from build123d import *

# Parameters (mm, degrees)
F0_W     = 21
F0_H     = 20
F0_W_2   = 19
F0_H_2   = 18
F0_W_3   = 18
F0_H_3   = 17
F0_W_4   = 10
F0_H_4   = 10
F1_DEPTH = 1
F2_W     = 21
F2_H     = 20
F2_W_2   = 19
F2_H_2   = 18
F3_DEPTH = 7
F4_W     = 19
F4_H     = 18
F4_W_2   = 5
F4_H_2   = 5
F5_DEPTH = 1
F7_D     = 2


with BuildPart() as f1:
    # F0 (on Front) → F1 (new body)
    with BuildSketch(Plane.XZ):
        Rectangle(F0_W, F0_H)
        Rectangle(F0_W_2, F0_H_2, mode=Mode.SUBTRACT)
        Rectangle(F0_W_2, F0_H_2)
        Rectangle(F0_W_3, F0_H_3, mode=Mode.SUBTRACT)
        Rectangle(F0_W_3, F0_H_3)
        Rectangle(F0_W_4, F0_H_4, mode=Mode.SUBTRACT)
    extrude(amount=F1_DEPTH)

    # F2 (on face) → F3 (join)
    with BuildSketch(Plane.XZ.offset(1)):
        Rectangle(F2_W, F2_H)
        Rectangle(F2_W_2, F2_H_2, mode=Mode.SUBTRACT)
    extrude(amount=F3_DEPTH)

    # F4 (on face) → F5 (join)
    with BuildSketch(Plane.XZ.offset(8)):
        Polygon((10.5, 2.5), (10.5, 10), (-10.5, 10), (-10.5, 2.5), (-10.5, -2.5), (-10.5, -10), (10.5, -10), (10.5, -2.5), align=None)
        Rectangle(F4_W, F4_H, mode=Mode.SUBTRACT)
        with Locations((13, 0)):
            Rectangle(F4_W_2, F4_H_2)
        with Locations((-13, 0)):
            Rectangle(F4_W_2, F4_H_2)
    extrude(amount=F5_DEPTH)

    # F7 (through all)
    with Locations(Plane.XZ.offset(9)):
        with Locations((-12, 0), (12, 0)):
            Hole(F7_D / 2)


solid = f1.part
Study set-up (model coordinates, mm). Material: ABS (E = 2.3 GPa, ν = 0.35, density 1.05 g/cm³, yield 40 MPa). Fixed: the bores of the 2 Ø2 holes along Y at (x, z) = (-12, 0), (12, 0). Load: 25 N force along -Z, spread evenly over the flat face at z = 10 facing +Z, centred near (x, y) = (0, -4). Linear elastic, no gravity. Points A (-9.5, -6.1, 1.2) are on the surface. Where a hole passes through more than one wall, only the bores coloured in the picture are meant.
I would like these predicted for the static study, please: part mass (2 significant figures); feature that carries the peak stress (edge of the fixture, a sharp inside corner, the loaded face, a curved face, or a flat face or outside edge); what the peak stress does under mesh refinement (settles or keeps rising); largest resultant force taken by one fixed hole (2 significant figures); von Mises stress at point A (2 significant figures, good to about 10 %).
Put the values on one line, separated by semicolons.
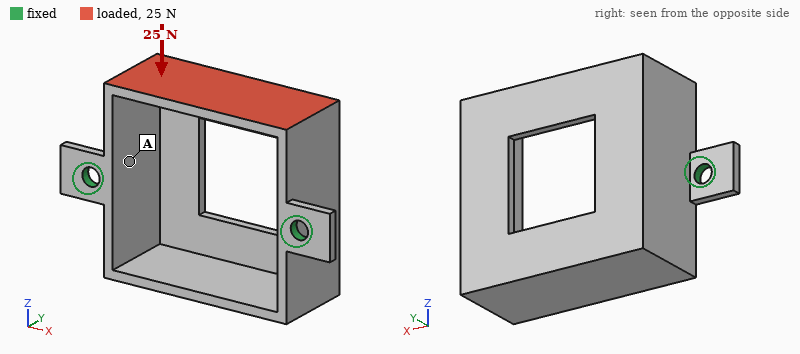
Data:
1.0 g; edge of the fixture; keeps rising; 13 N; 4.1 MPa
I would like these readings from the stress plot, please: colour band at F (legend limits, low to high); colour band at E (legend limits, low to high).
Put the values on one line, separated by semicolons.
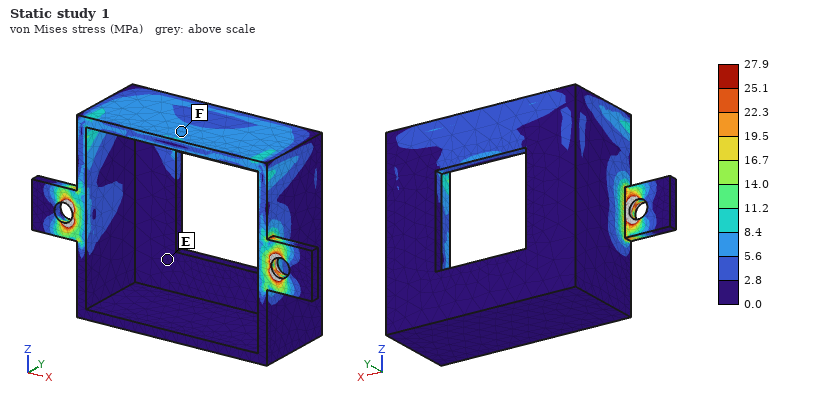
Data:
5.6 to 8.4 MPa; 0.0 to 2.8 MPa
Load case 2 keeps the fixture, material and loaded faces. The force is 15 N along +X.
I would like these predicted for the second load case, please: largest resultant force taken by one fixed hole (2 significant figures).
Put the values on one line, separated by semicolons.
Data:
9.3 N
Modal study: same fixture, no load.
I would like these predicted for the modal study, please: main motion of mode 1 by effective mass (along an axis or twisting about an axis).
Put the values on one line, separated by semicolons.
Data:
along Z
